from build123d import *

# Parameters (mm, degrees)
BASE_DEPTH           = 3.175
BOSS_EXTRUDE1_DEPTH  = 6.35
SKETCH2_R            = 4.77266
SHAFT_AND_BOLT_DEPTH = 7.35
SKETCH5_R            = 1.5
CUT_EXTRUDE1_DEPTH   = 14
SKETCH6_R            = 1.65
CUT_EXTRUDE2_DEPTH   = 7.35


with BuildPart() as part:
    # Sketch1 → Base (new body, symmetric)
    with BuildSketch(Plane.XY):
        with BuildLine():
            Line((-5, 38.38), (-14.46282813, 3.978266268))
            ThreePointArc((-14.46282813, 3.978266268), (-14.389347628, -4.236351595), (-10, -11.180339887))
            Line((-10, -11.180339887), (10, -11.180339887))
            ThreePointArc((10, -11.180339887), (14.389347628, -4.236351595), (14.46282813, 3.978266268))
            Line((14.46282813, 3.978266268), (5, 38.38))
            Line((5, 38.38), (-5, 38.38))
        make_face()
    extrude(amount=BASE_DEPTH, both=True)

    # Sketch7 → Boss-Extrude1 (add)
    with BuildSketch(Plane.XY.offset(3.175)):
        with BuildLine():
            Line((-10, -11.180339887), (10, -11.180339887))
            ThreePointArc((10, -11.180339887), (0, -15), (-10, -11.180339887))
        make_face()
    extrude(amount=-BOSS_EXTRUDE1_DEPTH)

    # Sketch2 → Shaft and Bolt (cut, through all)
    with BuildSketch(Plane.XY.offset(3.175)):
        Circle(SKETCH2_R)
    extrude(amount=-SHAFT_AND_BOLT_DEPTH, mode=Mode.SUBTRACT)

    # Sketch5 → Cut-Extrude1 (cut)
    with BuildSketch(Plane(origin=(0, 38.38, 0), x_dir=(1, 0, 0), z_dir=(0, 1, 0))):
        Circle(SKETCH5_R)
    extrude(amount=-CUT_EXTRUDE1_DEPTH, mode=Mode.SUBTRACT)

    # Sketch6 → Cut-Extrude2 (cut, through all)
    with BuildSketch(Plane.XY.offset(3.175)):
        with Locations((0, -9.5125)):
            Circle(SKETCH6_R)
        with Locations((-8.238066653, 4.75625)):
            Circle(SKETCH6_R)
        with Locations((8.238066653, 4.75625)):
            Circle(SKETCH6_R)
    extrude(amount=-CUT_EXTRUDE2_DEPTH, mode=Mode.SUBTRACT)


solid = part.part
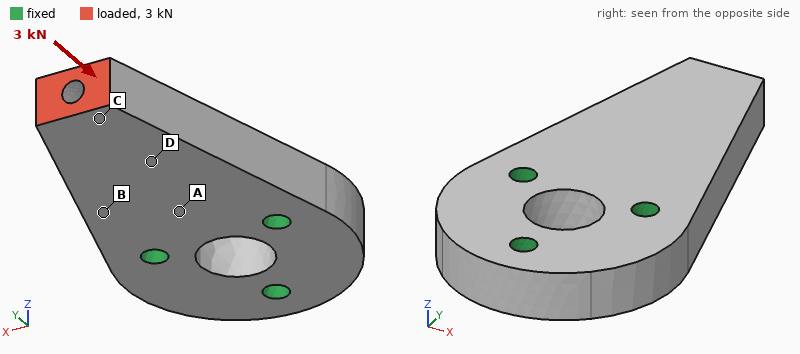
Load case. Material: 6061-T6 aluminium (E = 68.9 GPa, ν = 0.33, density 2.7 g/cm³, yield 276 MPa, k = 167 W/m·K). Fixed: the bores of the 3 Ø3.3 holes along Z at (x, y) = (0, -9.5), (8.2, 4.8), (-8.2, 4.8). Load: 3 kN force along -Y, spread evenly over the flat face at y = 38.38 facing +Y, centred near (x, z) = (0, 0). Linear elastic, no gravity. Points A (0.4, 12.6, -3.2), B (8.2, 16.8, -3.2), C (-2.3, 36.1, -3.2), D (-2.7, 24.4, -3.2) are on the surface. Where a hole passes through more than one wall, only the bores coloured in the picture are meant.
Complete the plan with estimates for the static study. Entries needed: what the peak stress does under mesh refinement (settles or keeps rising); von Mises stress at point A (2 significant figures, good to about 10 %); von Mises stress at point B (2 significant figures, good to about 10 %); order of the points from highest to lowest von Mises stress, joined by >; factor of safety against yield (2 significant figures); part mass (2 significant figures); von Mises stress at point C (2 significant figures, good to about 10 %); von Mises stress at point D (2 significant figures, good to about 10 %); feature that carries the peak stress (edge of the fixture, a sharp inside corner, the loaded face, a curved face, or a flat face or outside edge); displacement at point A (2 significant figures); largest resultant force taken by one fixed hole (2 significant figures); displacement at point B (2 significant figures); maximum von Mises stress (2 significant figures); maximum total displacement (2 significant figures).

settles
15 MPa
23 MPa
C > D > B > A
4.5
18 g
49 MPa
29 MPa
a curved face
3.3 µm
1.5 kN
3.9 µm
61 MPa
16 µm
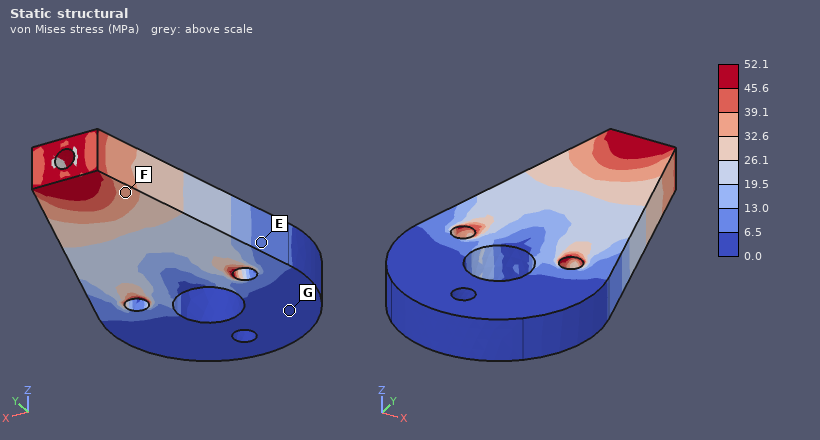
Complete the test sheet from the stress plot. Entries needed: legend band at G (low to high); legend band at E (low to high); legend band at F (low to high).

0.0 to 6.5 MPa
6.5 to 13.0 MPa
32.6 to 39.1 MPa
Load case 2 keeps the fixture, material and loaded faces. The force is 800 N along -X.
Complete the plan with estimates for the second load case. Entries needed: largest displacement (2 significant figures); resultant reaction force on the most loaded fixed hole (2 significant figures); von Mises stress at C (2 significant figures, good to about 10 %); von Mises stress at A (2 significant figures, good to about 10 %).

37 µm
1.4 kN
29 MPa
7.5 MPa
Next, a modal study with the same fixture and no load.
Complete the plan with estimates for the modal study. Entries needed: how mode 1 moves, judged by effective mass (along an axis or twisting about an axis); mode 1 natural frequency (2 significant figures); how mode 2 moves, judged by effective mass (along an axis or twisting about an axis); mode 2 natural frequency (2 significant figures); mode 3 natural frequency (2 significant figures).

along Z
5900 Hz
along X
18 kHz
22 kHz
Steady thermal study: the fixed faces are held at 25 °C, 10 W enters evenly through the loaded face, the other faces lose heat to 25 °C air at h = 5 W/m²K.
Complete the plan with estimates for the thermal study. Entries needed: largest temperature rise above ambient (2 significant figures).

20 K
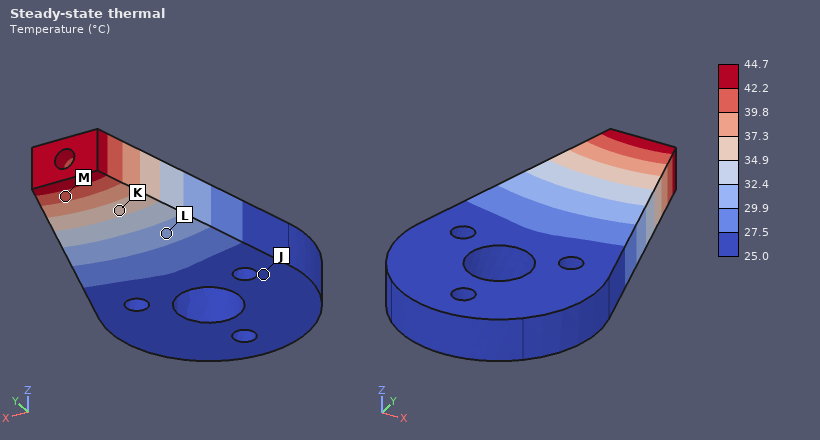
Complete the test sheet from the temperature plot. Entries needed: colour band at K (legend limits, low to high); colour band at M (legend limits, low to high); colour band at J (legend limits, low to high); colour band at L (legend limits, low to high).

34.9 to 37.3 °C
39.8 to 42.2 °C
25.0 to 27.5 °C
29.9 to 32.4 °C
